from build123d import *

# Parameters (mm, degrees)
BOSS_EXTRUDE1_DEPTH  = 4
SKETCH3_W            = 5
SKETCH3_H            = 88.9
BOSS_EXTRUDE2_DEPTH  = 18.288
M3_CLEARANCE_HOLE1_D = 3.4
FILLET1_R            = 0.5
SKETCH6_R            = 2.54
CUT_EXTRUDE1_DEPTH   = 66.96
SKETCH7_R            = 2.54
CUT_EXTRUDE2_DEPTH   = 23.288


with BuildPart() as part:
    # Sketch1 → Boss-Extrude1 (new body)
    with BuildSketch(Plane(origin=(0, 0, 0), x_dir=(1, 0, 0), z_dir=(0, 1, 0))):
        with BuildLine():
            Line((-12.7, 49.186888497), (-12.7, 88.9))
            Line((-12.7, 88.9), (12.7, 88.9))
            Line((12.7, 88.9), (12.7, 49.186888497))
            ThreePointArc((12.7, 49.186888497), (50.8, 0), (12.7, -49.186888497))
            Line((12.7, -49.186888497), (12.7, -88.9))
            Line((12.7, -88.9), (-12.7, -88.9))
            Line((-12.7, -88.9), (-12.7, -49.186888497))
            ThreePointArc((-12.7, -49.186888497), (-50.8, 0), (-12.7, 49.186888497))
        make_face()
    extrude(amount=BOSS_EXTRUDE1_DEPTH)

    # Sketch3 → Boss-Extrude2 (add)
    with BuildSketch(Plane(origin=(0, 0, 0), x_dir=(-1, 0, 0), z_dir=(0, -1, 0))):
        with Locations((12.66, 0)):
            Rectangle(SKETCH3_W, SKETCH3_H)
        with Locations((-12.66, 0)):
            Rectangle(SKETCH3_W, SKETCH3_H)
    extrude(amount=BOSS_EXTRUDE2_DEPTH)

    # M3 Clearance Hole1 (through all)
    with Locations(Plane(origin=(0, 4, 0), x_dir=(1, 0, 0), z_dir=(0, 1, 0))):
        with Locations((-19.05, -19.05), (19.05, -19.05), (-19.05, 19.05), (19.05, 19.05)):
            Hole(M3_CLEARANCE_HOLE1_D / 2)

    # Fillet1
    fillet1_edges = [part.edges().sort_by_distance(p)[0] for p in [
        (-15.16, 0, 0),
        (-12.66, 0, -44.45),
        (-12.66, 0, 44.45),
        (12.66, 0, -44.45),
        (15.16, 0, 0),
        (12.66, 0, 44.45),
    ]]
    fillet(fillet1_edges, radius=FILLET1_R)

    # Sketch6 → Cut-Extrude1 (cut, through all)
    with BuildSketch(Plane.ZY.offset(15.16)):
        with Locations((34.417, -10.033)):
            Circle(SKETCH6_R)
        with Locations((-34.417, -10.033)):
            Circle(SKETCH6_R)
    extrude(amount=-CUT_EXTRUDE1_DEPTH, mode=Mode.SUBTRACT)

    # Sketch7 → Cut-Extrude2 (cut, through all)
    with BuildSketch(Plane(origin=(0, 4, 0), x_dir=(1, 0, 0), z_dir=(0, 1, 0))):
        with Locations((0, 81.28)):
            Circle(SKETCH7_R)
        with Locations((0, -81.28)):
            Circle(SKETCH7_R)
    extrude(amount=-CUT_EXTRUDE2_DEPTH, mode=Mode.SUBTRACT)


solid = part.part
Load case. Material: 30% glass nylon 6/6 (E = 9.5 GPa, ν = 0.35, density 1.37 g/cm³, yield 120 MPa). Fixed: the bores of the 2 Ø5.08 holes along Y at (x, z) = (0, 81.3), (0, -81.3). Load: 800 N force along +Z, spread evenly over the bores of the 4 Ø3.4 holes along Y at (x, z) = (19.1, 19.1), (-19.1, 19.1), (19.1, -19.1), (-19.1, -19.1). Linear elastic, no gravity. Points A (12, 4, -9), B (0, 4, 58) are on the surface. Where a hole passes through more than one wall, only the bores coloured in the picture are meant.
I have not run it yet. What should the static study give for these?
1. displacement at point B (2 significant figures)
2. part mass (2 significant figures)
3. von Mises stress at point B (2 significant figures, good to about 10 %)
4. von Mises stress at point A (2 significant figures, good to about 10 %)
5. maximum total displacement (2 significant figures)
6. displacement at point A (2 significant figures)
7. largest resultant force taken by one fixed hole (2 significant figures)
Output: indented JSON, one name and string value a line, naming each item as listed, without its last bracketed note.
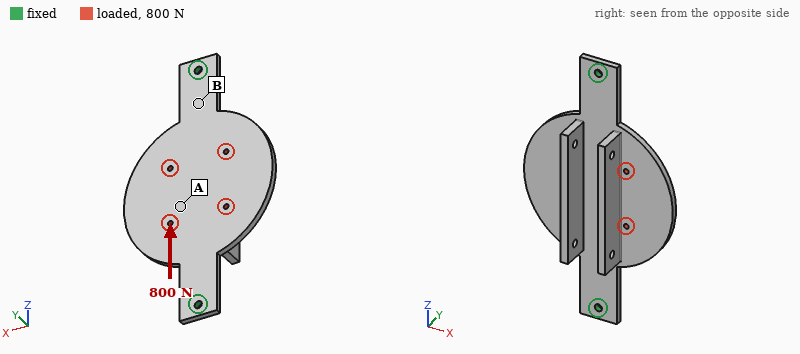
{
  "displacement at point B": "12 µm",
  "part mass": "76 g",
  "von Mises stress at point B": "3.7 MPa",
  "von Mises stress at point A": "1.2 MPa",
  "maximum total displacement": "28 µm",
  "displacement at point A": "25 µm",
  "largest resultant force taken by one fixed hole": "400 N"
}
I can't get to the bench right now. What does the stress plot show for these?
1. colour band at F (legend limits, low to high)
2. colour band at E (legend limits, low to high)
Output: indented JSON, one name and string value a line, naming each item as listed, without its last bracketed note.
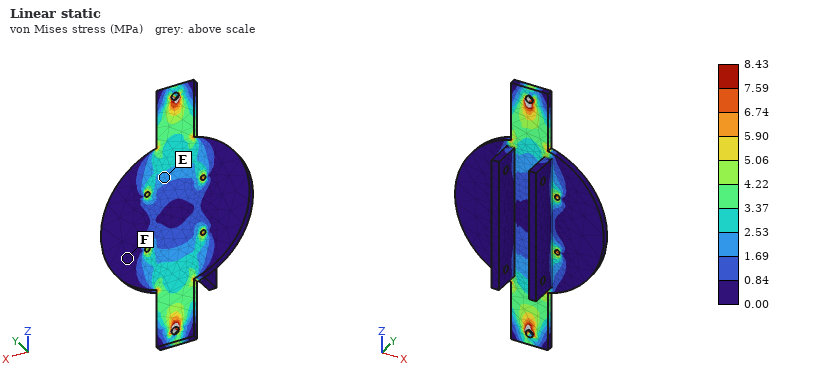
{
  "colour band at F": "0.00 to 0.84 MPa",
  "colour band at E": "1.69 to 2.53 MPa"
}
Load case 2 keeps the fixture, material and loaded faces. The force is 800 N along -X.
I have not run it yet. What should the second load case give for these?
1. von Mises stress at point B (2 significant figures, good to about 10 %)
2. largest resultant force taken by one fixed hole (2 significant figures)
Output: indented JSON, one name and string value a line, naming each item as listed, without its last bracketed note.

{
  "von Mises stress at point B": "9.5 MPa",
  "largest resultant force taken by one fixed hole": "400 N"
}
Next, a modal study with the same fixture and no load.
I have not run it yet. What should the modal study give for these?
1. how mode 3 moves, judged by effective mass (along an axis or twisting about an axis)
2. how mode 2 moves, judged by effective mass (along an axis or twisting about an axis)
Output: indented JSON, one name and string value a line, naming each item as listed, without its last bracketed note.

{
  "how mode 3 moves, judged by effective mass": "twisting about X",
  "how mode 2 moves, judged by effective mass": "along Y"
}
